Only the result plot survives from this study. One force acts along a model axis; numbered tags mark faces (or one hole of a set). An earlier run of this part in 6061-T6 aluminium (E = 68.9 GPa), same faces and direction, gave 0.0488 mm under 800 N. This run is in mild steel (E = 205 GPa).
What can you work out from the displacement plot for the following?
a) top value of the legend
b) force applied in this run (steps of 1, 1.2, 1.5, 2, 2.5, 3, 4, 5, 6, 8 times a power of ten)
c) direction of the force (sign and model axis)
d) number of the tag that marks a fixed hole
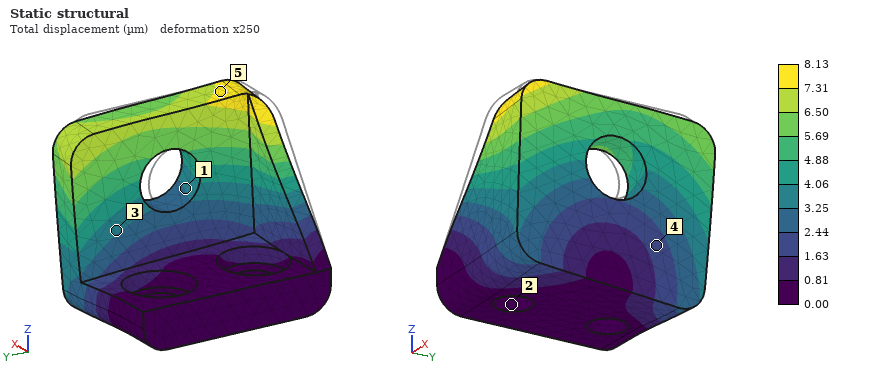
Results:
8.13 µm
400 N
+Y
2
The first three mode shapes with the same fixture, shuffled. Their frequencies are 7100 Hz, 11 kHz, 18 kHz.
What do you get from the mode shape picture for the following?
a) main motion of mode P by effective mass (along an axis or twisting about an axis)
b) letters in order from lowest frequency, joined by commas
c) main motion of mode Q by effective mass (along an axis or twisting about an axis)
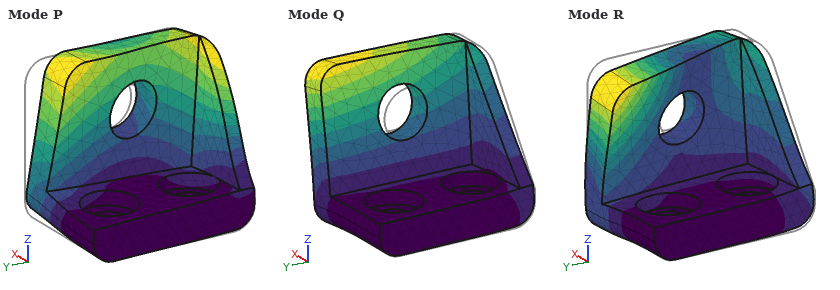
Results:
along Y
Q, P, R
along X
